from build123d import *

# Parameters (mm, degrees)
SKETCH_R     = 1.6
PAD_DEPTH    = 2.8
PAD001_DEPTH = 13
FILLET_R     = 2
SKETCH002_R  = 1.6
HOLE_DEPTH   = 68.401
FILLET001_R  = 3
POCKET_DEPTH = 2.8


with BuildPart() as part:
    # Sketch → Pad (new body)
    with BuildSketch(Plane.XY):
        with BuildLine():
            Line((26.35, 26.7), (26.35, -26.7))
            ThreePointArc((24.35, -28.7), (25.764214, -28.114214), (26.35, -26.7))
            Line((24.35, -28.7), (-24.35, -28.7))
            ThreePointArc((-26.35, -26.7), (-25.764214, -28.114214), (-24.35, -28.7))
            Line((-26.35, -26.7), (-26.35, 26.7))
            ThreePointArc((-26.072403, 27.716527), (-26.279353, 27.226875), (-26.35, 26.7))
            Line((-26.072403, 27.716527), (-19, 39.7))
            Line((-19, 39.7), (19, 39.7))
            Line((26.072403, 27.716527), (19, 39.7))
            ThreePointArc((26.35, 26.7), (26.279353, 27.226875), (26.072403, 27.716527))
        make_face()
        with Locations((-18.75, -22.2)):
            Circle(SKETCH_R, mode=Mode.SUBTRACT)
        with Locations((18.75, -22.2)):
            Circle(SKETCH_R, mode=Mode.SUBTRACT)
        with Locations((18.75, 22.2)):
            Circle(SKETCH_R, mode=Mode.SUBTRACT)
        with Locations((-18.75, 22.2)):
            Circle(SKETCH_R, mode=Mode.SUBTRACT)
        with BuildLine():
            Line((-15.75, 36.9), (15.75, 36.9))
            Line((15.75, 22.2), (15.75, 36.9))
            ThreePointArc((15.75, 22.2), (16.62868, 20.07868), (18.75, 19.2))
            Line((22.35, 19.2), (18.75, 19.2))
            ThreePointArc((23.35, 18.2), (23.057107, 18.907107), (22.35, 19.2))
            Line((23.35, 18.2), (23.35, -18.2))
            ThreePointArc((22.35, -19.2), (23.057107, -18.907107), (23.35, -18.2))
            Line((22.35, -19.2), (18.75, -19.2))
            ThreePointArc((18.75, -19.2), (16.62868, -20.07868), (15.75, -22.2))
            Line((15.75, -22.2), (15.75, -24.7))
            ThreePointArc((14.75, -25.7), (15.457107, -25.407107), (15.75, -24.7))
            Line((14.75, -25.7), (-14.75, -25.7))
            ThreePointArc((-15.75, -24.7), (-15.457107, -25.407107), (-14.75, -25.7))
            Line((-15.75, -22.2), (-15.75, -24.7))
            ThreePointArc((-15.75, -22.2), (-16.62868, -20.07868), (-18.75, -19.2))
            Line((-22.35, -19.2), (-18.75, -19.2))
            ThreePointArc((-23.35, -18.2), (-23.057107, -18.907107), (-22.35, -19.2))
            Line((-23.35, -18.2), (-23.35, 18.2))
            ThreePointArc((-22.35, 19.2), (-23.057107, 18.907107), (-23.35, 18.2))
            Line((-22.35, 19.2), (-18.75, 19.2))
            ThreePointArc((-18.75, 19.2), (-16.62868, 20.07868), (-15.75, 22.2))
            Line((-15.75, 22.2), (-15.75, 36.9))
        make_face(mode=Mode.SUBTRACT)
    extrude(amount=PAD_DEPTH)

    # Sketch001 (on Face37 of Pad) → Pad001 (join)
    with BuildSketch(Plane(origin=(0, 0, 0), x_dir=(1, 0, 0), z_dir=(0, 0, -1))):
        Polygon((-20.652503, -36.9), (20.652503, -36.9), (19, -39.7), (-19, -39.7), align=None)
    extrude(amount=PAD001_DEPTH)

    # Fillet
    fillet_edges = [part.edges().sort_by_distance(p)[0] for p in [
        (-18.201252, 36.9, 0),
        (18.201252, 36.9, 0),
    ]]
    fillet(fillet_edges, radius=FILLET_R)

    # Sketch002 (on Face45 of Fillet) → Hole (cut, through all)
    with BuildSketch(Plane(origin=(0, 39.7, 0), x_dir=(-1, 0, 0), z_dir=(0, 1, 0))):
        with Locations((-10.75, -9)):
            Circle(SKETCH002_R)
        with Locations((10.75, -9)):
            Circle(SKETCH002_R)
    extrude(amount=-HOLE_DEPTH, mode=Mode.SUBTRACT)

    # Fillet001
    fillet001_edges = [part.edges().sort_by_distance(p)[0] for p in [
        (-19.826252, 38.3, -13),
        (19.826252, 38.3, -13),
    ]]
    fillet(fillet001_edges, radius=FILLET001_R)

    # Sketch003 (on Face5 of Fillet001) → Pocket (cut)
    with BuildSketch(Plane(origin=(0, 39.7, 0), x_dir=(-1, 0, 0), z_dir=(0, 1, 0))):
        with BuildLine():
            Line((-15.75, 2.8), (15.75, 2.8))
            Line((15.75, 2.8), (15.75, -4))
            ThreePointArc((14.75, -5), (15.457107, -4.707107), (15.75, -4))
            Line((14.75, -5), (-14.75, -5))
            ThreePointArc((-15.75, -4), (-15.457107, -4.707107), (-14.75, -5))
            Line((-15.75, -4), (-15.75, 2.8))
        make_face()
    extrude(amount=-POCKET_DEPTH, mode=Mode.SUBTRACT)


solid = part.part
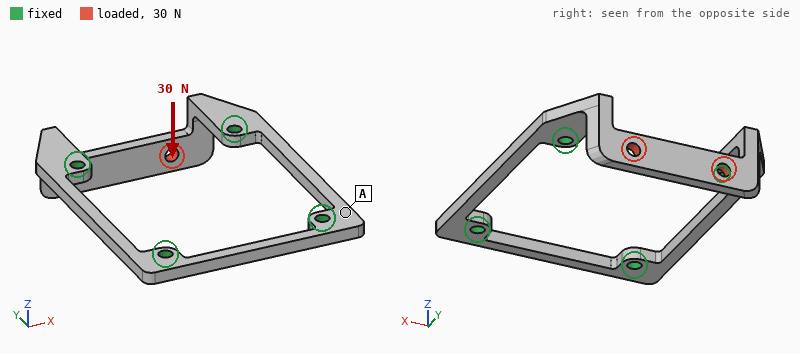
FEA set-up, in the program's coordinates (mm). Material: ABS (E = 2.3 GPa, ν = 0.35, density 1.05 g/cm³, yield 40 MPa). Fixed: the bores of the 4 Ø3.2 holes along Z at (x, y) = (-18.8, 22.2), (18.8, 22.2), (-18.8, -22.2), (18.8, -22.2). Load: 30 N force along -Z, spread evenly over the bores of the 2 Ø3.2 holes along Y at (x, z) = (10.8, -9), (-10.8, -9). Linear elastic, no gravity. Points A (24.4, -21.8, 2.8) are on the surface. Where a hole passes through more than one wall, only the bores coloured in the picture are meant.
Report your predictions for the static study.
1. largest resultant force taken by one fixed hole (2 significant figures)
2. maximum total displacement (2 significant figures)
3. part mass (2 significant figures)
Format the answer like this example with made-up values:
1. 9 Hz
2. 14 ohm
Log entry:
1. 16 N
2. 0.97 mm
3. 3.4 g
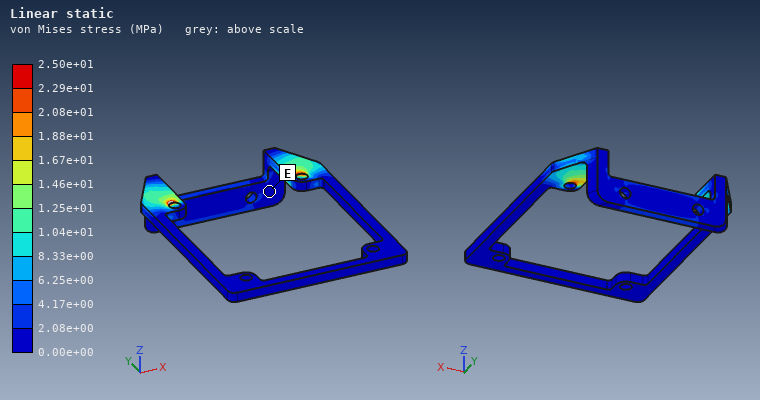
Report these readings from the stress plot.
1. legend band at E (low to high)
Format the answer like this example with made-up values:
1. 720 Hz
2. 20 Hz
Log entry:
1. 0.00e+00 to 2.08e+00 MPa
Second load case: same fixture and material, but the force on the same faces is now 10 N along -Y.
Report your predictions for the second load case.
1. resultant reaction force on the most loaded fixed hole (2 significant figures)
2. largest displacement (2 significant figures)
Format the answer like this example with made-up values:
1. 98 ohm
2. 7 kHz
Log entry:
1. 5.2 N
2. 0.61 mm
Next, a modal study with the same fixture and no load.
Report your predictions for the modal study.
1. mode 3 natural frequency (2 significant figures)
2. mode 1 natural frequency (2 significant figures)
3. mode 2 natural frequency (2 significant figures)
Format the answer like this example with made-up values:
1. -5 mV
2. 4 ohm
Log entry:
1. 1800 Hz
2. 730 Hz
3. 1500 Hz
